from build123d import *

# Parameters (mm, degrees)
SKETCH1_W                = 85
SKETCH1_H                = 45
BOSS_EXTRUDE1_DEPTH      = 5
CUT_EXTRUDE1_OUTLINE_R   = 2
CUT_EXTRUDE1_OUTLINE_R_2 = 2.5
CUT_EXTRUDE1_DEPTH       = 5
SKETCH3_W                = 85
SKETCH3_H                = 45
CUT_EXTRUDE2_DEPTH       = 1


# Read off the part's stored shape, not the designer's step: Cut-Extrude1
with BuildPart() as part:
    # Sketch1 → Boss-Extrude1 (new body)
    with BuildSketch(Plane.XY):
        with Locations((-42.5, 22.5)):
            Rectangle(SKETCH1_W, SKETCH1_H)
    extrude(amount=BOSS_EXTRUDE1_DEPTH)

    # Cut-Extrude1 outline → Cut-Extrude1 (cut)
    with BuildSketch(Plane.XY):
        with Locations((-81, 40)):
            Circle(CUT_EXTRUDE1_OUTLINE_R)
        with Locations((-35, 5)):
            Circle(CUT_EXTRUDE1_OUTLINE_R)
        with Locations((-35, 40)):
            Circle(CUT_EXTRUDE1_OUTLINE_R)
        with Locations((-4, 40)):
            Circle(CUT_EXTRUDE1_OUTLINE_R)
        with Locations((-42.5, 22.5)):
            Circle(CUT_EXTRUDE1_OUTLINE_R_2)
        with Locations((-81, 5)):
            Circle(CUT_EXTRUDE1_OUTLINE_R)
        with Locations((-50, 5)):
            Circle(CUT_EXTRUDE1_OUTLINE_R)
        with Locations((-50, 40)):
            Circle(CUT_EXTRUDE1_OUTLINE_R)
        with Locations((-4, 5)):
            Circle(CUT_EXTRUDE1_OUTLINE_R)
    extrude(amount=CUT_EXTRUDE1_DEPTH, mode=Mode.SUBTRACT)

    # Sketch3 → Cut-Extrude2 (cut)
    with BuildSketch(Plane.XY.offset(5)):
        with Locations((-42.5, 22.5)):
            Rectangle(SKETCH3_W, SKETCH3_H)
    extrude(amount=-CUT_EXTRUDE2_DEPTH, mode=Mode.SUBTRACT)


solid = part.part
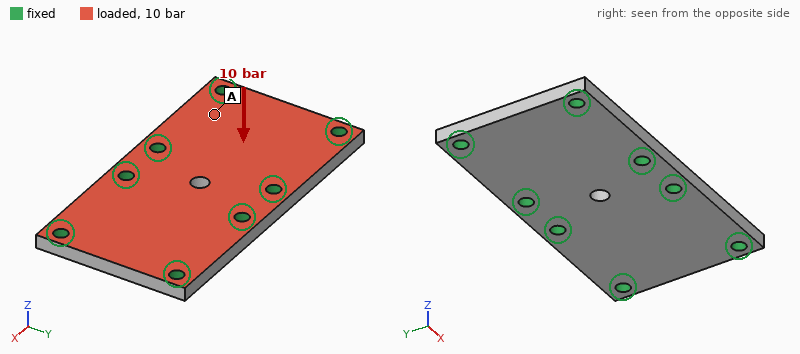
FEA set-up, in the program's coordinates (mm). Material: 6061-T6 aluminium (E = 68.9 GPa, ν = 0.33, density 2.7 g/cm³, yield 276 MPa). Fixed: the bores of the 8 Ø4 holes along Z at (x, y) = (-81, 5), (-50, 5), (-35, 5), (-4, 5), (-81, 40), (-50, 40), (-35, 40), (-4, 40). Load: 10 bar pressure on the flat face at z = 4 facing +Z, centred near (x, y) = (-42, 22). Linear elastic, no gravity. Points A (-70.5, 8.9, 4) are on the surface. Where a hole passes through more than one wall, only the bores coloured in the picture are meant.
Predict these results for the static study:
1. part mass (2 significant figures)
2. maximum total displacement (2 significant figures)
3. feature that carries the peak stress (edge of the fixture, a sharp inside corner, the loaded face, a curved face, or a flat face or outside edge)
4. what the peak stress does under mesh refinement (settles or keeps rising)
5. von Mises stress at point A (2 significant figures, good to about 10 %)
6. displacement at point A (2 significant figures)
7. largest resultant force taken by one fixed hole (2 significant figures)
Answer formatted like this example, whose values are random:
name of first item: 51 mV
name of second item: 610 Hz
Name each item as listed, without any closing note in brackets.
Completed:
part mass: 40 g
maximum total displacement: 20 µm
feature that carries the peak stress: edge of the fixture
what the peak stress does under mesh refinement: keeps rising
von Mises stress at point A: 12 MPa
displacement at point A: 10 µm
largest resultant force taken by one fixed hole: 500 N
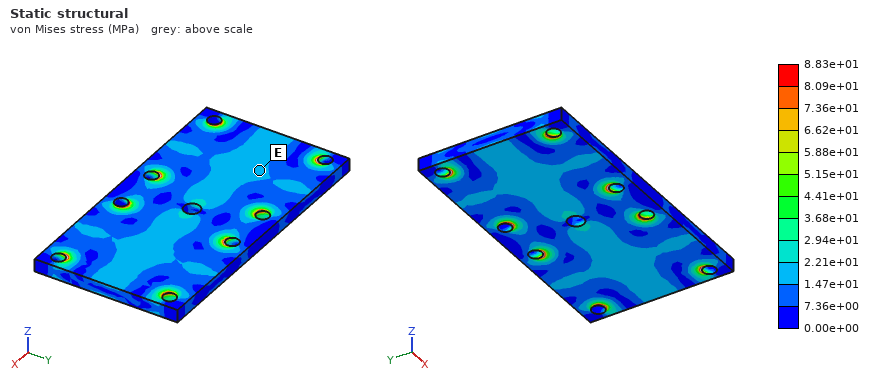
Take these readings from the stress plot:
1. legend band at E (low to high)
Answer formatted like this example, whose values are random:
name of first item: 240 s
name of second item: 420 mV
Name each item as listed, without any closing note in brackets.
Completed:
legend band at E: 1.47e+01 to 2.21e+01 MPa
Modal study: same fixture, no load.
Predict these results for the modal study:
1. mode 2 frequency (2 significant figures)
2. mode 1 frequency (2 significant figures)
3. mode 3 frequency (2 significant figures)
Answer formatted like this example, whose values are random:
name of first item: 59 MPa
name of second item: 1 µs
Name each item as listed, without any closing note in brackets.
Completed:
mode 2 frequency: 13 kHz
mode 1 frequency: 13 kHz
mode 3 frequency: 19 kHz
